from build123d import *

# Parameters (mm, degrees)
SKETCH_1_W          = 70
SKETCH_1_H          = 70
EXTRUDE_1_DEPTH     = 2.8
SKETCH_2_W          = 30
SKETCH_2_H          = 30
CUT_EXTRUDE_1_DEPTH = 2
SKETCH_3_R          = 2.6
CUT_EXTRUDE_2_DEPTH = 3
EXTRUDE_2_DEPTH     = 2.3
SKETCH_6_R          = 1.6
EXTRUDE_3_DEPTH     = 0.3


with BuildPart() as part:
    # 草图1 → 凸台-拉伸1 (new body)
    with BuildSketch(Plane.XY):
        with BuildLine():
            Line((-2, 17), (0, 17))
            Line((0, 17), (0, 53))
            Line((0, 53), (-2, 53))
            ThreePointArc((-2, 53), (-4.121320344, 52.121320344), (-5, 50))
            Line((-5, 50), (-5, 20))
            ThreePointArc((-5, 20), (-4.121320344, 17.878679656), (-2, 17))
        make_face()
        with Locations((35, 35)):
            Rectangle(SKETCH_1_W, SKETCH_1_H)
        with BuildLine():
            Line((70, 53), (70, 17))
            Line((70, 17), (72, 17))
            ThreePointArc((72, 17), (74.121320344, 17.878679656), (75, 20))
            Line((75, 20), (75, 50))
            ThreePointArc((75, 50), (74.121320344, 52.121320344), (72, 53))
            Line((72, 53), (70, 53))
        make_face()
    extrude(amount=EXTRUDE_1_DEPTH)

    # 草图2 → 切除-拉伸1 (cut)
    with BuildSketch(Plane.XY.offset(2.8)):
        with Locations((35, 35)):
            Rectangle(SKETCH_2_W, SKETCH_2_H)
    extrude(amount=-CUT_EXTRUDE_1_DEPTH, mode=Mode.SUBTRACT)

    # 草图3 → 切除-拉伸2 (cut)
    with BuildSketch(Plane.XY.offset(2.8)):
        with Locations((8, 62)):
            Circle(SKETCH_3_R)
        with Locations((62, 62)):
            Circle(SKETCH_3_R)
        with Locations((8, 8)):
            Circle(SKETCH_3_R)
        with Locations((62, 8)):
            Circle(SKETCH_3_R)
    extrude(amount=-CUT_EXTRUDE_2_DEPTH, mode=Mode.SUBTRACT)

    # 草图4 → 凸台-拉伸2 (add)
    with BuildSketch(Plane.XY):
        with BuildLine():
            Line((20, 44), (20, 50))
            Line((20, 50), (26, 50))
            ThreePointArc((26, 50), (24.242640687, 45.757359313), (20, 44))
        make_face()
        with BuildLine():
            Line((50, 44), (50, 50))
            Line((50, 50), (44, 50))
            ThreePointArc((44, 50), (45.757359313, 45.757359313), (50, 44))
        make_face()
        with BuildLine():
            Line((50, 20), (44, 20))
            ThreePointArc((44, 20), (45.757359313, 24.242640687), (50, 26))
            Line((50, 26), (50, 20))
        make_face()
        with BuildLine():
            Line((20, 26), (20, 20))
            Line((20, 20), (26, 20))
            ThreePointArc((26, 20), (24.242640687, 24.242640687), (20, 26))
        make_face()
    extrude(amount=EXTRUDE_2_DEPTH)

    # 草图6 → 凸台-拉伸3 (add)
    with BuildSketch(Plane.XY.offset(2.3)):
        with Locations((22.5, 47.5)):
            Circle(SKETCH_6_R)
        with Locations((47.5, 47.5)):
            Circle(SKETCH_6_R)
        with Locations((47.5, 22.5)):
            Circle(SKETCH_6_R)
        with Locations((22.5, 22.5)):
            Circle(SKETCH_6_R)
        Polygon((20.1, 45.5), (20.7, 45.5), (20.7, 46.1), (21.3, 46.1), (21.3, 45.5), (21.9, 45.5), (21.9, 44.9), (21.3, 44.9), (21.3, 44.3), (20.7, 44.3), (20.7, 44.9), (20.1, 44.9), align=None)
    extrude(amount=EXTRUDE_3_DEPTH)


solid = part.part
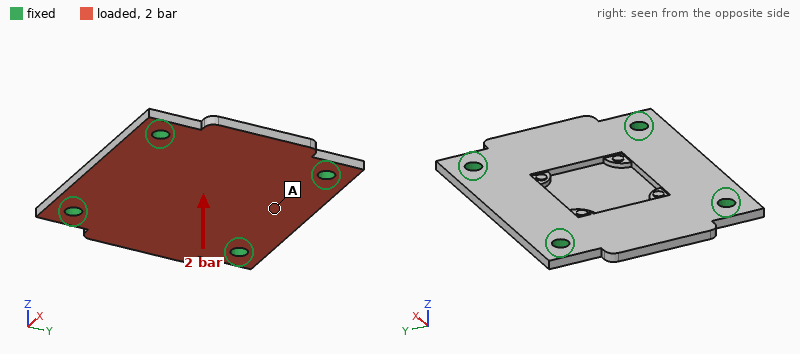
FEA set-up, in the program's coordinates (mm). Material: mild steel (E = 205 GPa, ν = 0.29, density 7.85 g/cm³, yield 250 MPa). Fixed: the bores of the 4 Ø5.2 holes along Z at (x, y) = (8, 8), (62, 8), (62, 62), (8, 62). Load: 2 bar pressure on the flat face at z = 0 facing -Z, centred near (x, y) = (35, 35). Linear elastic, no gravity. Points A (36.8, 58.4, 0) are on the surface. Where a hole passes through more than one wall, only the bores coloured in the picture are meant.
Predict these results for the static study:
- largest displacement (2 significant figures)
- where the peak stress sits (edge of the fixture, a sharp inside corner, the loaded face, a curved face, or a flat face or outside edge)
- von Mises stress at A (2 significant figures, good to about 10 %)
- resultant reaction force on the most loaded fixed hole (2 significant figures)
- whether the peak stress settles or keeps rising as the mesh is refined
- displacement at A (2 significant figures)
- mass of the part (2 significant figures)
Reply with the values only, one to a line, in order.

52 µm
edge of the fixture
22 MPa
290 N
keeps rising
17 µm
100 g
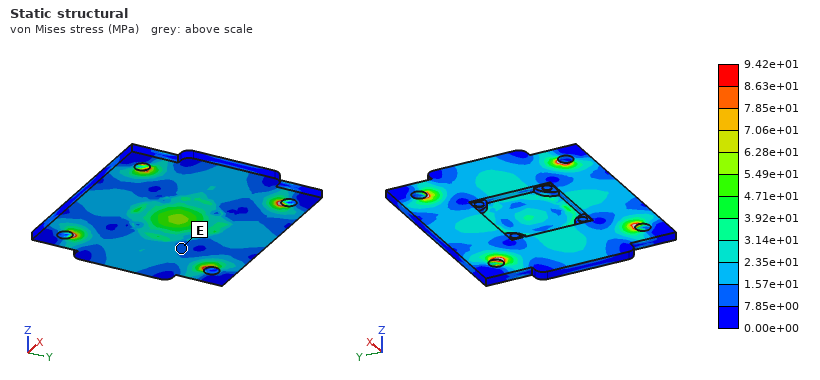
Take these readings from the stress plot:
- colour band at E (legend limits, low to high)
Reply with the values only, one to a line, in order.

7.85e+00 to 1.57e+01 MPa
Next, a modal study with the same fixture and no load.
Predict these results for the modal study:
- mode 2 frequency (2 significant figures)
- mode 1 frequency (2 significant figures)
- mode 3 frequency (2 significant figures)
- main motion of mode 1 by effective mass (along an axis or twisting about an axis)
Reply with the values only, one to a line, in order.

5000 Hz
4200 Hz
5100 Hz
along Z
